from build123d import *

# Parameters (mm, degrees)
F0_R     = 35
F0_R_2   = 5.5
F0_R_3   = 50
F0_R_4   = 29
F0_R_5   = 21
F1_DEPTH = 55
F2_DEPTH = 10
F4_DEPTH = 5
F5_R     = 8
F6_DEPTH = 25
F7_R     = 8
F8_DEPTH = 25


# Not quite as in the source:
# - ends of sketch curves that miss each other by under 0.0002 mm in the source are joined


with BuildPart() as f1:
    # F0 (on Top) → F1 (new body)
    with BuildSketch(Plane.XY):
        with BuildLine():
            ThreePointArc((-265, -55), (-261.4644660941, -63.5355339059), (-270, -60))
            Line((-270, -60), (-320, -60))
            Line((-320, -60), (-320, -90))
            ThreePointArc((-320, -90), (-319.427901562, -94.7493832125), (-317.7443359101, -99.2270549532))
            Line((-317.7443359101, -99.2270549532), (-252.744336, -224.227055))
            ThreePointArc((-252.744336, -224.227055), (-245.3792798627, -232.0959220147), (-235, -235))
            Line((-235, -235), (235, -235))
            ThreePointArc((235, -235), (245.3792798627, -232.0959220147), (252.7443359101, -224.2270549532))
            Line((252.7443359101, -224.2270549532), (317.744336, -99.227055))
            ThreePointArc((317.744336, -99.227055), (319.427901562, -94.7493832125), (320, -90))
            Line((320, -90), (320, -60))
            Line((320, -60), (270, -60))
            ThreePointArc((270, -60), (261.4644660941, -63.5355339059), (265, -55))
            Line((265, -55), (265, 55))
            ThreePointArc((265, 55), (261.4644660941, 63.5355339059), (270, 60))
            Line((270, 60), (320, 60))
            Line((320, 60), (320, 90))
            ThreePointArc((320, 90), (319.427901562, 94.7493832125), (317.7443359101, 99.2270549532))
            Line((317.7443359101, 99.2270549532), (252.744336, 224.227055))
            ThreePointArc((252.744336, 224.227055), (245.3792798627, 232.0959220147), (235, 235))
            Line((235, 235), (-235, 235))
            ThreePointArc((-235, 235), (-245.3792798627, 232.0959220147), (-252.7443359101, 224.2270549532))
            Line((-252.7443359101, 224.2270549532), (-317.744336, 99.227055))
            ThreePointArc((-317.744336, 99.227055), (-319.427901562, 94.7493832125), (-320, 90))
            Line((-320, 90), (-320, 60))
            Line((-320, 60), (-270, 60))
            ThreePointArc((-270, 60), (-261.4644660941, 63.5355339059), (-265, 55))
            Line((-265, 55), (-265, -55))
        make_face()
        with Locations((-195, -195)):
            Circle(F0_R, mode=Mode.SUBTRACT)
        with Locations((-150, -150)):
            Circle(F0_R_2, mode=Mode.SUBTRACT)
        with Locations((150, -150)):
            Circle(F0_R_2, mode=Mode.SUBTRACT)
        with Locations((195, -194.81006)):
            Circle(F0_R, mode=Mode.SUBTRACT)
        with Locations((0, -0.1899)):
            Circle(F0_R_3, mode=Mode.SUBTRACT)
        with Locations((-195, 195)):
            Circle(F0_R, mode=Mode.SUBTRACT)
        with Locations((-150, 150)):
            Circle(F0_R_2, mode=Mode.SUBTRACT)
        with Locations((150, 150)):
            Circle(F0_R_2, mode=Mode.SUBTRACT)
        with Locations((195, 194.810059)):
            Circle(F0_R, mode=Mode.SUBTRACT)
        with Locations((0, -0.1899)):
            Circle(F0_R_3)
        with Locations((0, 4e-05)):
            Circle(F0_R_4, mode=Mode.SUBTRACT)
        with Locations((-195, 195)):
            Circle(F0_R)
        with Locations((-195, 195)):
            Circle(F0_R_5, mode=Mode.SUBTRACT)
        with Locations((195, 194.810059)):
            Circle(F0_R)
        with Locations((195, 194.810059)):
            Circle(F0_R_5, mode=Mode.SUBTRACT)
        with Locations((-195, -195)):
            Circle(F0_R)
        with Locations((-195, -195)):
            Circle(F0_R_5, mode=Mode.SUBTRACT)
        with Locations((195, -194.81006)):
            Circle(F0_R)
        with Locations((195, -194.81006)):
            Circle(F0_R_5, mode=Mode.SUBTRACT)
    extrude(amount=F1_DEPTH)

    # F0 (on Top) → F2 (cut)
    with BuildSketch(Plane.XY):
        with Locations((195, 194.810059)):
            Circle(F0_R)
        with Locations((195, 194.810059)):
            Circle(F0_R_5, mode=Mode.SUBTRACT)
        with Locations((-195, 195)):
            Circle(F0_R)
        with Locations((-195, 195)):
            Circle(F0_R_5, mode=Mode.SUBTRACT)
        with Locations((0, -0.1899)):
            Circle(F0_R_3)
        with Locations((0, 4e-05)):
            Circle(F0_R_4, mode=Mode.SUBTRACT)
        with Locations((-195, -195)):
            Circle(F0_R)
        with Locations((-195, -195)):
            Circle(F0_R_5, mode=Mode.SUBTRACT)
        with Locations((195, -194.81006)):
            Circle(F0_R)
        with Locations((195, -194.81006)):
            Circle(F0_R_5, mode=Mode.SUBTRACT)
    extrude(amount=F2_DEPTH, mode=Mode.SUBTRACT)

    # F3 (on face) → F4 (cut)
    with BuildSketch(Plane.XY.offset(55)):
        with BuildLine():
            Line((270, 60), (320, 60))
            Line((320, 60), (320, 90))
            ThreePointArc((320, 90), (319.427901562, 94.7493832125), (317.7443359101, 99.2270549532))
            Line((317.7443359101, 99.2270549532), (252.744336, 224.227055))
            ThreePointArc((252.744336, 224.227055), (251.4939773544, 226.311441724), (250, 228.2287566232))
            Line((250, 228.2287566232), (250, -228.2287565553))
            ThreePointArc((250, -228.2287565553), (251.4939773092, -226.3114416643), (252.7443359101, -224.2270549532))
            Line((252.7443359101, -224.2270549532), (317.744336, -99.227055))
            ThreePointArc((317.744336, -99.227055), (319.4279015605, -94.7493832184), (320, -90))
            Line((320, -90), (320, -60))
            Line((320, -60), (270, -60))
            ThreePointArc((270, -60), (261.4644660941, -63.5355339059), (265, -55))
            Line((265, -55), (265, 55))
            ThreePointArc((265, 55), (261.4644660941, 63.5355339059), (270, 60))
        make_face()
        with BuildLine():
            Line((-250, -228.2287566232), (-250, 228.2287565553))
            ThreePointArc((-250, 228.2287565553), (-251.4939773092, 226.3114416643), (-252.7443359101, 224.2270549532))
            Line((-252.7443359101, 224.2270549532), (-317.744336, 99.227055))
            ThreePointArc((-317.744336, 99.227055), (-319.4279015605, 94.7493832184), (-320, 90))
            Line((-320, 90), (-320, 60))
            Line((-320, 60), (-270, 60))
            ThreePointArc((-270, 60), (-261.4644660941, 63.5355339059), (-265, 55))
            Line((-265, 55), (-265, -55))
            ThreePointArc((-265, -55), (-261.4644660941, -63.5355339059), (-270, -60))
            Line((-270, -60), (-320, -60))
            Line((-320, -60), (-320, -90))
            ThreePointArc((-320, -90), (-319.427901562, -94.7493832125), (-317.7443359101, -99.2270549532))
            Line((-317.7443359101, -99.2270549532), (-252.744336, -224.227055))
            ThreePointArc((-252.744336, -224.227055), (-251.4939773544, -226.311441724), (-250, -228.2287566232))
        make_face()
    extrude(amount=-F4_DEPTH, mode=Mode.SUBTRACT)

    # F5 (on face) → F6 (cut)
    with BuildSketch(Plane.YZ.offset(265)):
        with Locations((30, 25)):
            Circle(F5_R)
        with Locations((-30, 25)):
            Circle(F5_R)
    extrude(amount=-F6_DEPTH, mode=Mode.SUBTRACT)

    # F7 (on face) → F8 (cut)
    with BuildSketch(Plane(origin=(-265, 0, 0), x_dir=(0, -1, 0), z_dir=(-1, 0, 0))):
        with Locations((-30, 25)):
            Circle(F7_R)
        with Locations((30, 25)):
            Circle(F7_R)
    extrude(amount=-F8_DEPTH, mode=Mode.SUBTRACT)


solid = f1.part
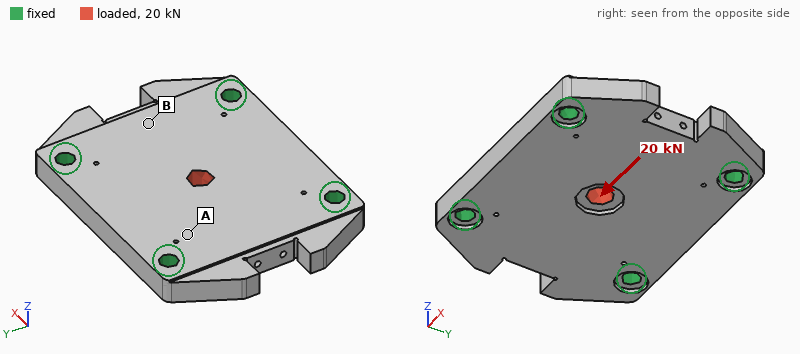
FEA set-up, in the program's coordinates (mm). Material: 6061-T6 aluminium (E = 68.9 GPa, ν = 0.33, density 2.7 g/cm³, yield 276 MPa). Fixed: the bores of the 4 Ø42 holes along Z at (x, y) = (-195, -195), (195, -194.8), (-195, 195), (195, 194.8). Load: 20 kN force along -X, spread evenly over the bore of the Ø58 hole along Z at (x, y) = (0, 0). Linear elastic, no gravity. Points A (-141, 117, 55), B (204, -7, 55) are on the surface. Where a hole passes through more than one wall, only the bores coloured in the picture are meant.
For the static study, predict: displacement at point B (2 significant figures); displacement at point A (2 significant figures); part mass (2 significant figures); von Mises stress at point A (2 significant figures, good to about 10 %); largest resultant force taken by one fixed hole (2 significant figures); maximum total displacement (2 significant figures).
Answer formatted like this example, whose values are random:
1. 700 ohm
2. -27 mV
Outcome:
1. 2.7 µm
2. 1.7 µm
3. 37 kg
4. 0.95 MPa
5. 5.5 kN
6. 5.3 µm
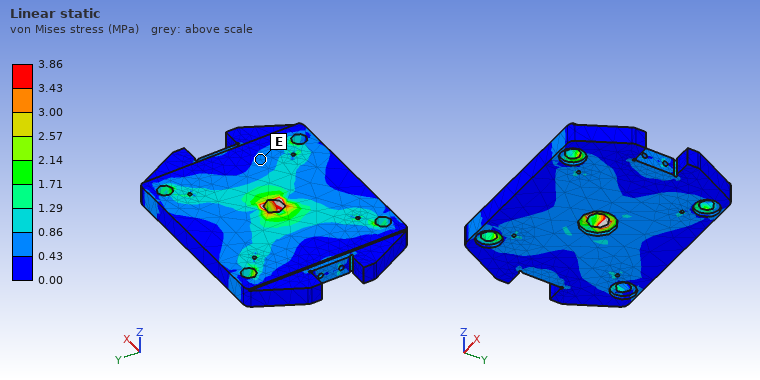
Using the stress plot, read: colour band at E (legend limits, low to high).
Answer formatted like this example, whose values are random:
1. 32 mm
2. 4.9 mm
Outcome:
1. 0.43 to 0.86 MPa
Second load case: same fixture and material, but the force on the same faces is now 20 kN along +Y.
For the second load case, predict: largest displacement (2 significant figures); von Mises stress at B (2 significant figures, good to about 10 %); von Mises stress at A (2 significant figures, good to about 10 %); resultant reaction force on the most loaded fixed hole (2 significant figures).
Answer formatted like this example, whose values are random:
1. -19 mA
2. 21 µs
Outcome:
1. 5.3 µm
2. 0.25 MPa
3. 1.00 MPa
4. 5.7 kN
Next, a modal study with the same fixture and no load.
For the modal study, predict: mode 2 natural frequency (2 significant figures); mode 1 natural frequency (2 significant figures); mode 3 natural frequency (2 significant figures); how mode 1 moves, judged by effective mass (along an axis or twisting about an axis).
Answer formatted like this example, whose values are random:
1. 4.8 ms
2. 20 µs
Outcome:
1. 1600 Hz
2. 1100 Hz
3. 1600 Hz
4. along Z
